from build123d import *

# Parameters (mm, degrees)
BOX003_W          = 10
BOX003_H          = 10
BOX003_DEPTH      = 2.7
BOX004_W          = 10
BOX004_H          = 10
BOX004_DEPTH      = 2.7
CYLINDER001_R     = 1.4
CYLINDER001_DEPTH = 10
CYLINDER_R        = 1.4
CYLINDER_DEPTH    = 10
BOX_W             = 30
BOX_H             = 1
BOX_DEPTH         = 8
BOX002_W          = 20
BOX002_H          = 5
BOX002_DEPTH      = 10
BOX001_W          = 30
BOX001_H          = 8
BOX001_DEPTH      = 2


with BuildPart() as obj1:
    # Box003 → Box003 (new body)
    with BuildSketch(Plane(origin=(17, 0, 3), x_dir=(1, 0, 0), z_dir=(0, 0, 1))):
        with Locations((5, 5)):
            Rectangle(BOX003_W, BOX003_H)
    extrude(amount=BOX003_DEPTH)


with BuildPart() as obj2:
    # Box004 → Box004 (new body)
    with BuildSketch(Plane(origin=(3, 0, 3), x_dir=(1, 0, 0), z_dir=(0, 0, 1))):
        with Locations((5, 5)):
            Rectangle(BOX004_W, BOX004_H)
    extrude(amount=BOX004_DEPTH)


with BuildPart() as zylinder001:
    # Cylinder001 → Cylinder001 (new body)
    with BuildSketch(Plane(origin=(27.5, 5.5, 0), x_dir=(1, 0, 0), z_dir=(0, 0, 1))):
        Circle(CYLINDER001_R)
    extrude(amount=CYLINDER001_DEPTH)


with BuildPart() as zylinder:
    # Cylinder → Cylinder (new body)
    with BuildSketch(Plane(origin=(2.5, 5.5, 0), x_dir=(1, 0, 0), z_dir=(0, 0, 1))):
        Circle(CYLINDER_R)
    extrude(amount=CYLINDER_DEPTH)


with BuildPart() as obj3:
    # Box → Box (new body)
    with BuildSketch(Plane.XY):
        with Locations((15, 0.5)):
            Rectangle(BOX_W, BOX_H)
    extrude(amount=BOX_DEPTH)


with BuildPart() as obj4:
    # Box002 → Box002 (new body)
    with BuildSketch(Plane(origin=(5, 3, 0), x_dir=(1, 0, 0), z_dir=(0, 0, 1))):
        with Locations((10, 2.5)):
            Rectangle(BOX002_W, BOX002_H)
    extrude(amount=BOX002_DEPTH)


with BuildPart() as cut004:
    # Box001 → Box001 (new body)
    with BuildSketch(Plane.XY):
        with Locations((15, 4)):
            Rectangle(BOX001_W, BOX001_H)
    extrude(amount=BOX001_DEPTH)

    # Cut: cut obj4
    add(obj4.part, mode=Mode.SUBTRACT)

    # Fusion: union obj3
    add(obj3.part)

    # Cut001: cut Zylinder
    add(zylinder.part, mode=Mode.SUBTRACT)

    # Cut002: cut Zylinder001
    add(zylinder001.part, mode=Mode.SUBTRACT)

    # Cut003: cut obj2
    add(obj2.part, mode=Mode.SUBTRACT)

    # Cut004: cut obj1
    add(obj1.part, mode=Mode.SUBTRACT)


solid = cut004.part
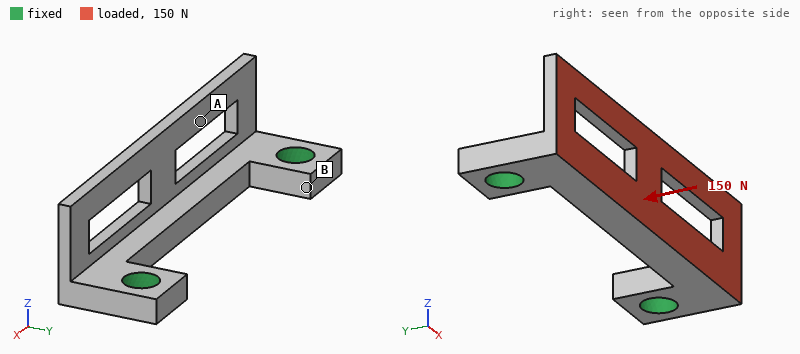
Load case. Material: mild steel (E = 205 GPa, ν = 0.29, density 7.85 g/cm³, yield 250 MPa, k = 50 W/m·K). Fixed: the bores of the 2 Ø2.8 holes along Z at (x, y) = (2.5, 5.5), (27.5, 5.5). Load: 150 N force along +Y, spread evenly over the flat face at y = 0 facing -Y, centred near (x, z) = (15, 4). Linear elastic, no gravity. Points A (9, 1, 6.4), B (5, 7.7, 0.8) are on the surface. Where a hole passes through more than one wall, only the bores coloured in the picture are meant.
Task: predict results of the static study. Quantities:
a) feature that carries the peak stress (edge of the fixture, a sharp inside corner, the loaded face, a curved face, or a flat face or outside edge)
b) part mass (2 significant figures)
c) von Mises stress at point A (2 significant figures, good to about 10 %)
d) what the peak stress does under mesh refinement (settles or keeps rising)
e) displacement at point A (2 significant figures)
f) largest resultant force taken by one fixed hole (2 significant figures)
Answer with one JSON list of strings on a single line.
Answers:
["a sharp inside corner", "3.0 g", "41 MPa", "keeps rising", "32 µm", "83 N"]
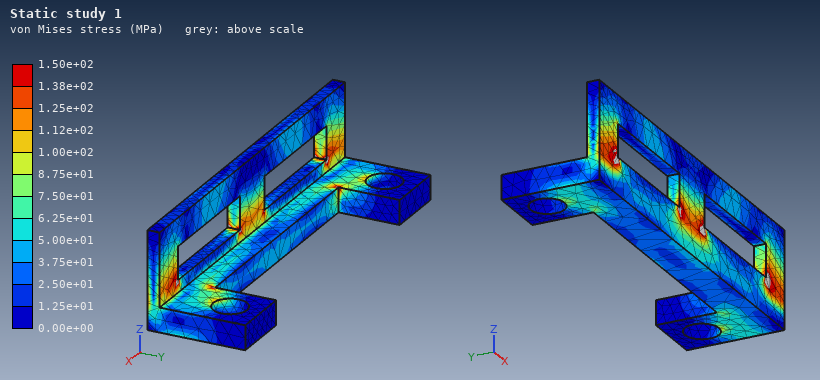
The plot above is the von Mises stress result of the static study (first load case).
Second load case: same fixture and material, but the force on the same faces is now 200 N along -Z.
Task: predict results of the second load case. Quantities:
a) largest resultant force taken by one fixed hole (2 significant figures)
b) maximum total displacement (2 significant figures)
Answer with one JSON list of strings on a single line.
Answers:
["100 N", "25 µm"]
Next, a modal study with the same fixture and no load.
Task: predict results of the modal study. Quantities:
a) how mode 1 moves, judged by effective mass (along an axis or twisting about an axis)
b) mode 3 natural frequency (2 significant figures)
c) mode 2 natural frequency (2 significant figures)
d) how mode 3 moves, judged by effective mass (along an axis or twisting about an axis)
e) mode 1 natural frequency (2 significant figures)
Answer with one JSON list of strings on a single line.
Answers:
["along Y", "17 kHz", "14 kHz", "along Z", "9300 Hz"]
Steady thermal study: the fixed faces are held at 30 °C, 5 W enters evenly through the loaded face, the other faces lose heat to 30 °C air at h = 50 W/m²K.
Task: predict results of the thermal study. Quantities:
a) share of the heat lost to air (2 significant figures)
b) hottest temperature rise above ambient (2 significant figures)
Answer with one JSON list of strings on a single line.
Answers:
["13 %", "50 K"]
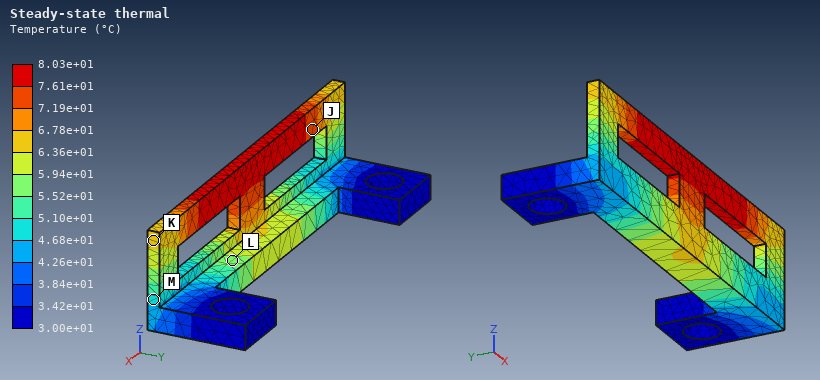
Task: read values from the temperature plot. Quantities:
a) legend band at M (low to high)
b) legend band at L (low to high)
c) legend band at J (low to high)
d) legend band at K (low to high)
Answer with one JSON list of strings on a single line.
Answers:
["4.68e+01 to 5.10e+01 °C", "5.52e+01 to 5.94e+01 °C", "7.19e+01 to 7.61e+01 °C", "6.36e+01 to 6.78e+01 °C"]
